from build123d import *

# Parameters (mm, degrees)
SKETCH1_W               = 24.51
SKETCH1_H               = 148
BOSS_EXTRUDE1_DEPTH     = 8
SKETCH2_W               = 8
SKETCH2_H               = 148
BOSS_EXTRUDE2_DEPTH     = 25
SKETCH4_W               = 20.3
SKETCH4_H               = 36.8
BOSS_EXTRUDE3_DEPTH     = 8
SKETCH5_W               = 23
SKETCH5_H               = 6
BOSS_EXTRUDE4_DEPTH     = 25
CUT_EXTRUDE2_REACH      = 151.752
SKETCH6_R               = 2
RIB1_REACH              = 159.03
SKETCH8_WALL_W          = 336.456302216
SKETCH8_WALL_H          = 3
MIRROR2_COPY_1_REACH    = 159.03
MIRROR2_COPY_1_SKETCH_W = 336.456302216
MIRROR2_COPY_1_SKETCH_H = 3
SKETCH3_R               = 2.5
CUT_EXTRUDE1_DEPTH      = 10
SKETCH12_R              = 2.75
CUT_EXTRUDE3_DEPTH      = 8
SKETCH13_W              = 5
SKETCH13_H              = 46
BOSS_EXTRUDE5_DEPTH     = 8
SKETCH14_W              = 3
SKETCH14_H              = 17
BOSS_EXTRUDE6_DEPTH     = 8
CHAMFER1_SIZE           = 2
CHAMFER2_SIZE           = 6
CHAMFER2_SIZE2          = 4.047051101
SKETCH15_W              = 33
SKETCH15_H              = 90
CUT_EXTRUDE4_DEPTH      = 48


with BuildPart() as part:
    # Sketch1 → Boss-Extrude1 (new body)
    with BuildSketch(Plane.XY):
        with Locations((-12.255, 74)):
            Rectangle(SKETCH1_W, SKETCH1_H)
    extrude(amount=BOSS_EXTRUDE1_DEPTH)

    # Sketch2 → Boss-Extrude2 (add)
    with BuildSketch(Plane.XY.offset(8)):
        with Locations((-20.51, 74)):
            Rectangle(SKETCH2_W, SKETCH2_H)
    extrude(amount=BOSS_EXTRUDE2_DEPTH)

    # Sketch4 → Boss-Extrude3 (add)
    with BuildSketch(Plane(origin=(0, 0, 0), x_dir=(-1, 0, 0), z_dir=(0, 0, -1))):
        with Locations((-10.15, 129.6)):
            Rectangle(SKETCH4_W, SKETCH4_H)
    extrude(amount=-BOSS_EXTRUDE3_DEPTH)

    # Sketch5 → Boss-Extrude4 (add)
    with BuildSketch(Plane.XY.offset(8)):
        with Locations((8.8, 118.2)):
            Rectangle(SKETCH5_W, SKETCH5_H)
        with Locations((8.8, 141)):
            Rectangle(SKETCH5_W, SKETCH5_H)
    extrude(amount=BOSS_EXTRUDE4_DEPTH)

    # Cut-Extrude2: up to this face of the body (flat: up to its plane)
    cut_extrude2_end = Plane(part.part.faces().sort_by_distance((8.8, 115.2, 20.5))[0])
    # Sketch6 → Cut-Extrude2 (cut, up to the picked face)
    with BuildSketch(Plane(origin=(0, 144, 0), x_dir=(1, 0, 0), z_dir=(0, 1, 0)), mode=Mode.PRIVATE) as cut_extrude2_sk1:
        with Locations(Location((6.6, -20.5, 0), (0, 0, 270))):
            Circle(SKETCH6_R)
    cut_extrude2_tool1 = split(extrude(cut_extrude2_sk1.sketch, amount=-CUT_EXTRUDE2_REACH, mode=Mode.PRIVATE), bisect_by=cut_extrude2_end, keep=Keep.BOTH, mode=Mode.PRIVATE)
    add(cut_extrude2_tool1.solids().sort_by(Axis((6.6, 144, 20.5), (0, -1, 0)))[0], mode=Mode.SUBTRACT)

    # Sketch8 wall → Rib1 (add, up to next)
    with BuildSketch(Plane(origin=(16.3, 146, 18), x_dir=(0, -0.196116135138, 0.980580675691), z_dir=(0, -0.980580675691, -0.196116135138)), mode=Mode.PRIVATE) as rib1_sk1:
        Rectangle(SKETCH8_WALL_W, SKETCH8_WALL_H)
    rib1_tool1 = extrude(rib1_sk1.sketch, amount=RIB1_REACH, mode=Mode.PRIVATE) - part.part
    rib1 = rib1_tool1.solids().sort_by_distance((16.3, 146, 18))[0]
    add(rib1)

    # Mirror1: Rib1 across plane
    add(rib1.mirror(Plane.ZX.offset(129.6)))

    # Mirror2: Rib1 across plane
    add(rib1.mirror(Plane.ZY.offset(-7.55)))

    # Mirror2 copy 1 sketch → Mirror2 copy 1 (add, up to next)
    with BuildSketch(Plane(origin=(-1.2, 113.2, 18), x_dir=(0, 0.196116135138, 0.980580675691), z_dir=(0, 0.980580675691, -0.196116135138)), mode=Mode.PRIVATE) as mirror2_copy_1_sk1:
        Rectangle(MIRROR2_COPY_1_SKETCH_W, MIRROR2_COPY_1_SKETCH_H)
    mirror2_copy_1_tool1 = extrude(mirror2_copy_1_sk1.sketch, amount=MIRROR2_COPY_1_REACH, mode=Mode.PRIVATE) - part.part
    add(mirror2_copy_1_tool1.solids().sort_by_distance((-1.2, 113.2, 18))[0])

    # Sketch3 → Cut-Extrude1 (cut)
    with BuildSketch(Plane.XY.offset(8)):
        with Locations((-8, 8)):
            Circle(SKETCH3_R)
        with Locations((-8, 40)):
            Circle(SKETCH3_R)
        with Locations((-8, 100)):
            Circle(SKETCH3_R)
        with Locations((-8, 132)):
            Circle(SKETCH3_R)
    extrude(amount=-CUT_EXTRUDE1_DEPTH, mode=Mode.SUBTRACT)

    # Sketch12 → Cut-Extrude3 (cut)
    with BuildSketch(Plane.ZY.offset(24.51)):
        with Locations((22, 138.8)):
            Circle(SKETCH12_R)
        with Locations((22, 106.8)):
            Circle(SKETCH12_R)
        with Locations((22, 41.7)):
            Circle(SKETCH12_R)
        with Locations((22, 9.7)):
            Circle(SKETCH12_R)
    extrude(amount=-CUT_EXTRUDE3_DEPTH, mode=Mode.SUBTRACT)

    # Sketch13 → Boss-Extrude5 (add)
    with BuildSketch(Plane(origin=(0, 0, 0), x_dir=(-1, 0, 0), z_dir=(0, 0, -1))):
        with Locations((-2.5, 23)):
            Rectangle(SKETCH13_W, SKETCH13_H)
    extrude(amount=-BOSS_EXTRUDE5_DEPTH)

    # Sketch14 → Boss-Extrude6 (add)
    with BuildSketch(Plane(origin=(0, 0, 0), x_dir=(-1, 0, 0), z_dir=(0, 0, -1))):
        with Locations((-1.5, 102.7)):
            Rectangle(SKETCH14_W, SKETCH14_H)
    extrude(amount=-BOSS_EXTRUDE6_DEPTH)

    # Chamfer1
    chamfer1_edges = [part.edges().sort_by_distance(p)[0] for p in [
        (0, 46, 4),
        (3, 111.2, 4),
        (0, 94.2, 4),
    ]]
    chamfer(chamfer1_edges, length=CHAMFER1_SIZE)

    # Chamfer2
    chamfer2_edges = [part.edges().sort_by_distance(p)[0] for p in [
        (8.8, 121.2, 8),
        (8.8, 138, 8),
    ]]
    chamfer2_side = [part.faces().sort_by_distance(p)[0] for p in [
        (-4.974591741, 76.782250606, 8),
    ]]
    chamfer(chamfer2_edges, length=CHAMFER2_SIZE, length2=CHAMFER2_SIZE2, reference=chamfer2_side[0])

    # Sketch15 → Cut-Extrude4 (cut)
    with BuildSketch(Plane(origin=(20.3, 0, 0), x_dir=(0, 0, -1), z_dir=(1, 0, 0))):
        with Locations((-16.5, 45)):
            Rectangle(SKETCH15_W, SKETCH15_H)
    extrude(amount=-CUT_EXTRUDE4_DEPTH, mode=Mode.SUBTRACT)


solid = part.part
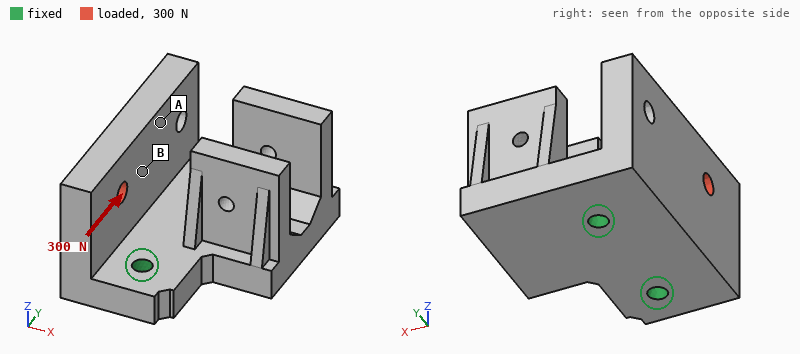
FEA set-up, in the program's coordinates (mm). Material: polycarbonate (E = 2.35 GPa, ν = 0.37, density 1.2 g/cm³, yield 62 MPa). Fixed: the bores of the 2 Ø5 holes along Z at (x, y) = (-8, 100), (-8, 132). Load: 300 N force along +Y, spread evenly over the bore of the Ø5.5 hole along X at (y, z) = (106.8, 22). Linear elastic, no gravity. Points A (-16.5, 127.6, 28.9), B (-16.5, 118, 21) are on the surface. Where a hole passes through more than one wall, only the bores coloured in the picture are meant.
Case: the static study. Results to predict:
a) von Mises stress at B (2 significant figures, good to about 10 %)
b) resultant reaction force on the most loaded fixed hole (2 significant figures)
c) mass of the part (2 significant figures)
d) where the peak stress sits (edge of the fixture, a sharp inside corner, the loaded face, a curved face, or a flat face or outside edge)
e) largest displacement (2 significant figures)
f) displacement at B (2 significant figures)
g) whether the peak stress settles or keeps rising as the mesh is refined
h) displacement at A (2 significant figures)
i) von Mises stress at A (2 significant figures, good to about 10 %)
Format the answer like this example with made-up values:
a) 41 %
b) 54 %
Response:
a) 2.2 MPa
b) 240 N
c) 44 g
d) edge of the fixture
e) 0.12 mm
f) 0.061 mm
g) keeps rising
h) 0.082 mm
i) 0.93 MPa
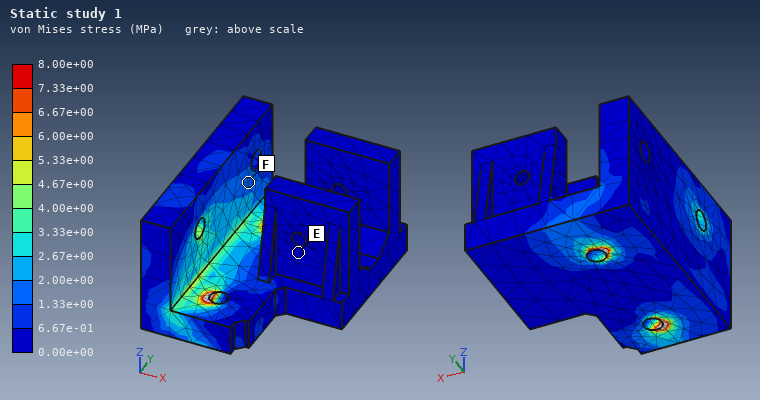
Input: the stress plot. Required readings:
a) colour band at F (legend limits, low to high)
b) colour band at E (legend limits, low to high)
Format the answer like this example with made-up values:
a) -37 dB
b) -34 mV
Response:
a) 1.33e+00 to 2.00e+00 MPa
b) 0.00e+00 to 6.67e-01 MPa
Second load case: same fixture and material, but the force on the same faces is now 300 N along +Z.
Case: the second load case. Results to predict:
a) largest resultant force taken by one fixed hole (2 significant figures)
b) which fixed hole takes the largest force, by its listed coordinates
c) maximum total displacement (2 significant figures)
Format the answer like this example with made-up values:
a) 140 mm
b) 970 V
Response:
a) 230 N
b) (-8, 100)
c) 0.22 mm
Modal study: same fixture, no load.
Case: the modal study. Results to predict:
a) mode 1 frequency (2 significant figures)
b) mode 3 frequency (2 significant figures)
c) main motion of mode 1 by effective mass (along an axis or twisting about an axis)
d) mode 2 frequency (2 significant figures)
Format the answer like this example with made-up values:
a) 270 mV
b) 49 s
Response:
a) 1100 Hz
b) 1600 Hz
c) along X
d) 1400 Hz
